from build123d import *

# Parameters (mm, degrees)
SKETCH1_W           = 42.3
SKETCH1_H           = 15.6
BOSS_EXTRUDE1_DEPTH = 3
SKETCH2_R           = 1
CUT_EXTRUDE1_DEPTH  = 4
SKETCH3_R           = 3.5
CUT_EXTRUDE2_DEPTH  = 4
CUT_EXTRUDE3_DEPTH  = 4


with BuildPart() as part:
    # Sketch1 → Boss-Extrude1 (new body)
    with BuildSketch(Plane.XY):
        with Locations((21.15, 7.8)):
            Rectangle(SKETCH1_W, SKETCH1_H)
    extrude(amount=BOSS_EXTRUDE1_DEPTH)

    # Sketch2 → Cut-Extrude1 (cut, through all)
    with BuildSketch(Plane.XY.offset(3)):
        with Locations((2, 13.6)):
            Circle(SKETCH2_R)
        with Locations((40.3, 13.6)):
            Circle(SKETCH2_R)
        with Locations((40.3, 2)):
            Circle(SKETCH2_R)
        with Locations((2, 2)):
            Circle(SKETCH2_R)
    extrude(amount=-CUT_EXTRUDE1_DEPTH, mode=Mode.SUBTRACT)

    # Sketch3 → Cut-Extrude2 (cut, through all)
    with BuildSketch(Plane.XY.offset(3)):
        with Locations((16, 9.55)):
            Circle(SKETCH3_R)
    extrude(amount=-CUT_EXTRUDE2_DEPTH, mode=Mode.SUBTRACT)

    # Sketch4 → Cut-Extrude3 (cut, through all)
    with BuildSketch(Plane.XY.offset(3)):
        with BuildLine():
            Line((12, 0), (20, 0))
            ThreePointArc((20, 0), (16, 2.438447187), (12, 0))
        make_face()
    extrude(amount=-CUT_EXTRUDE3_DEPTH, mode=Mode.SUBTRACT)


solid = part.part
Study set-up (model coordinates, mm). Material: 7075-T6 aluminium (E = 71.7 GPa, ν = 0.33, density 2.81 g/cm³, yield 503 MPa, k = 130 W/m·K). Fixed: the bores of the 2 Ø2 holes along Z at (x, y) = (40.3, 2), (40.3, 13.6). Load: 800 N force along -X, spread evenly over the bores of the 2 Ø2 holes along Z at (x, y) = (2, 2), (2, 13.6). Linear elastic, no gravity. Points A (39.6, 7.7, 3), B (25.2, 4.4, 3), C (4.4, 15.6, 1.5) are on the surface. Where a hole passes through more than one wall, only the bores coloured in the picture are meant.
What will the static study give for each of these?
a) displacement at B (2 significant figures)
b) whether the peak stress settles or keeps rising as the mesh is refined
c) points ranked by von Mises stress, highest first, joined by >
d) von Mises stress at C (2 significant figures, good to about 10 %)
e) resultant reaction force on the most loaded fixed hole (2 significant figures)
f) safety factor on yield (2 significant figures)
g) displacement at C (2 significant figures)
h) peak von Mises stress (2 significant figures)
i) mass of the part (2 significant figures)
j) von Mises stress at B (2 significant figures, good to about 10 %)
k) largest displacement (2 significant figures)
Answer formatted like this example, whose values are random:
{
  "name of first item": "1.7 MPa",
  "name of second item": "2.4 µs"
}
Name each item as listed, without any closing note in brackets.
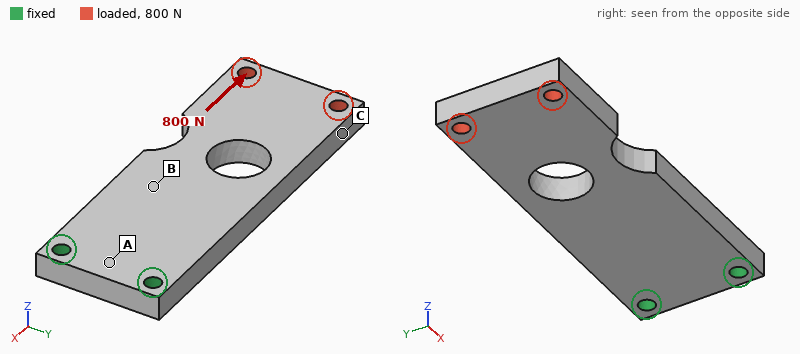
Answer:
{
  "displacement at B": "4.1 µm",
  "whether the peak stress settles or keeps rising as the mesh is refined": "settles",
  "points ranked by von Mises stress, highest first, joined by >": "C > B > A",
  "von Mises stress at C": "39 MPa",
  "resultant reaction force on the most loaded fixed hole": "410 N",
  "safety factor on yield": "6.2",
  "displacement at C": "13 µm",
  "peak von Mises stress": "81 MPa",
  "mass of the part": "5.0 g",
  "von Mises stress at B": "19 MPa",
  "largest displacement": "15 µm"
}
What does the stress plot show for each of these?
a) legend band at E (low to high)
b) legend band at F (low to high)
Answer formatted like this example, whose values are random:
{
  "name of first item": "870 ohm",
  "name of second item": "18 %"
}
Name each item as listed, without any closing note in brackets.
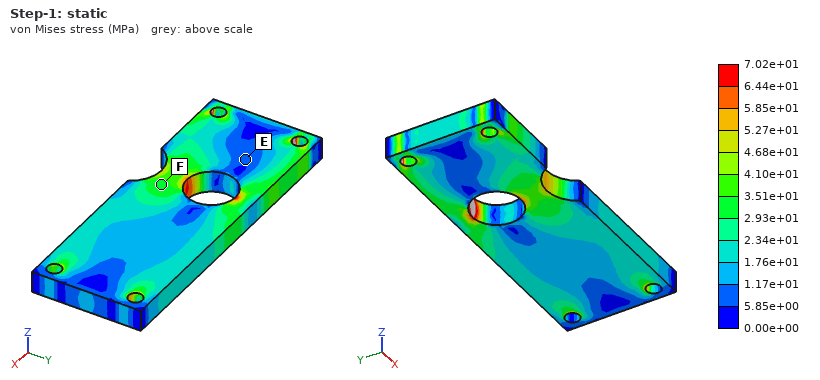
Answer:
{
  "legend band at E": "5.85e+00 to 1.17e+01 MPa",
  "legend band at F": "2.93e+01 to 3.51e+01 MPa"
}
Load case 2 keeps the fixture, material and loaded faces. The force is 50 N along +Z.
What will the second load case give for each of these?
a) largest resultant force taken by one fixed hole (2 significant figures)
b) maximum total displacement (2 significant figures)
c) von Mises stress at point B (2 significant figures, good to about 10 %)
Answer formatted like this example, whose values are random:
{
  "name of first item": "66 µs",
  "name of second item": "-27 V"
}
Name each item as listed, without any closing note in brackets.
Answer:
{
  "largest resultant force taken by one fixed hole": "25 N",
  "maximum total displacement": "0.46 mm",
  "von Mises stress at point B": "50 MPa"
}
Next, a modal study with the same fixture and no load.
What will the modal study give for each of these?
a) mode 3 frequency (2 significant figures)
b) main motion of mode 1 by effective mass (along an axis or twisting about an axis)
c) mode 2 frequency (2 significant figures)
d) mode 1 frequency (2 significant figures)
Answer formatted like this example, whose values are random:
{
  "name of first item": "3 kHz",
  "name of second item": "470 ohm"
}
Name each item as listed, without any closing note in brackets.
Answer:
{
  "mode 3 frequency": "7400 Hz",
  "main motion of mode 1 by effective mass": "along Z",
  "mode 2 frequency": "7100 Hz",
  "mode 1 frequency": "1500 Hz"
}
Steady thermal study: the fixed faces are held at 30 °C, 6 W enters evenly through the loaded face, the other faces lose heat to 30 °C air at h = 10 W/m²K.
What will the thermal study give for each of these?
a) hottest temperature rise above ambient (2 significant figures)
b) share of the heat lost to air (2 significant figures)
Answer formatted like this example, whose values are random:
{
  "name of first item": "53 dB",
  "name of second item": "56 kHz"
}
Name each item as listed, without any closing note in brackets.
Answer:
{
  "hottest temperature rise above ambient": "48 K",
  "share of the heat lost to air": "5.8 %"
}
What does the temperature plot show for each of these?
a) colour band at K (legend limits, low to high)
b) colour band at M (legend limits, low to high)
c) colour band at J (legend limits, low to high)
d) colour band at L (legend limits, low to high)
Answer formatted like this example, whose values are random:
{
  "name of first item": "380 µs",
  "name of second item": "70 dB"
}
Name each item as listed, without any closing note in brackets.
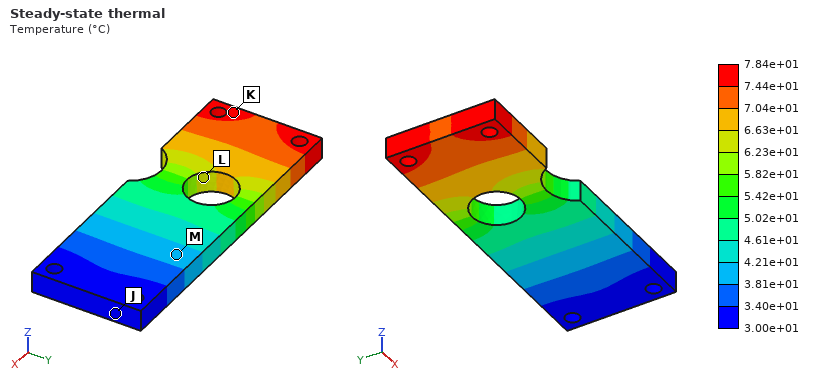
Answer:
{
  "colour band at K": "7.44e+01 to 7.84e+01 °C",
  "colour band at M": "3.81e+01 to 4.21e+01 °C",
  "colour band at J": "3.00e+01 to 3.40e+01 °C",
  "colour band at L": "6.23e+01 to 6.63e+01 °C"
}
